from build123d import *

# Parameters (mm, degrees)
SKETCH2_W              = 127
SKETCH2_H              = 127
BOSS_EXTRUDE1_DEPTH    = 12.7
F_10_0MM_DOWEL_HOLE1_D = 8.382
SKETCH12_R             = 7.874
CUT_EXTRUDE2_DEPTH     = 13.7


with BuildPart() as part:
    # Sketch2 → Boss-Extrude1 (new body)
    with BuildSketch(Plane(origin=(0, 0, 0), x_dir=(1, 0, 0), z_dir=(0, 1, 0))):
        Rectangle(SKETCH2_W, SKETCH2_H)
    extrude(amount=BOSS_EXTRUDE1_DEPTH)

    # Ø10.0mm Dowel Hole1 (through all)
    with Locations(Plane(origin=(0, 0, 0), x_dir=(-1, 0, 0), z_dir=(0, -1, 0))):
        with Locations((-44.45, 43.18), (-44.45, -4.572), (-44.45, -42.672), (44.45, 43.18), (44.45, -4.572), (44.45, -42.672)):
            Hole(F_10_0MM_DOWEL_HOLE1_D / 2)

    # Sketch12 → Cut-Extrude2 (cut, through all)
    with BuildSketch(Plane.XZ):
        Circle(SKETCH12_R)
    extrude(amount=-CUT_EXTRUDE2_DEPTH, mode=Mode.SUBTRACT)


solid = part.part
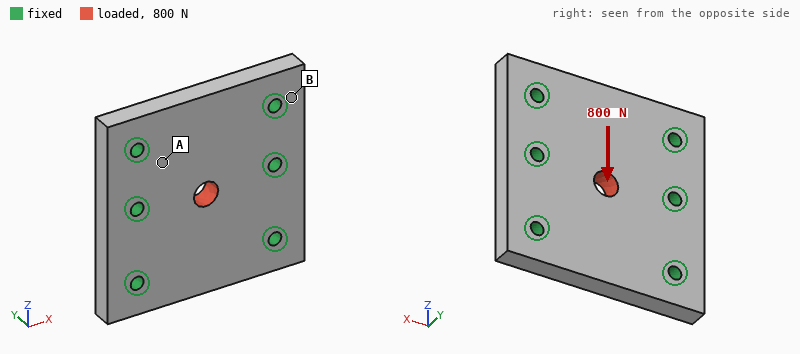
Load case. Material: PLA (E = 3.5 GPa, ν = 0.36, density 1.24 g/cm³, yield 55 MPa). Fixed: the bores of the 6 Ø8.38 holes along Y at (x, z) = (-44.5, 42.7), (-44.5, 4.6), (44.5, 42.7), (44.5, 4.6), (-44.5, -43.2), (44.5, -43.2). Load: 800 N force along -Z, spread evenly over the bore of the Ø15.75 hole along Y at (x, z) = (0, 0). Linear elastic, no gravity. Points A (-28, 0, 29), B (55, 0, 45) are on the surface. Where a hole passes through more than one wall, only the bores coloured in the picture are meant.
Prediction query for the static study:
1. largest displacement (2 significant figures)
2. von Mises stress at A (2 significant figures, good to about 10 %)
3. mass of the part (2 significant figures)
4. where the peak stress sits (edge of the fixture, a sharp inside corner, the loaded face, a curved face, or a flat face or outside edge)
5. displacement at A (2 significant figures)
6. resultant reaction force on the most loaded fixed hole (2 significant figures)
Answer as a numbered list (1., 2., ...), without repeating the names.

1. 13 µm
2. 0.60 MPa
3. 250 g
4. the loaded face
5. 3.7 µm
6. 160 N
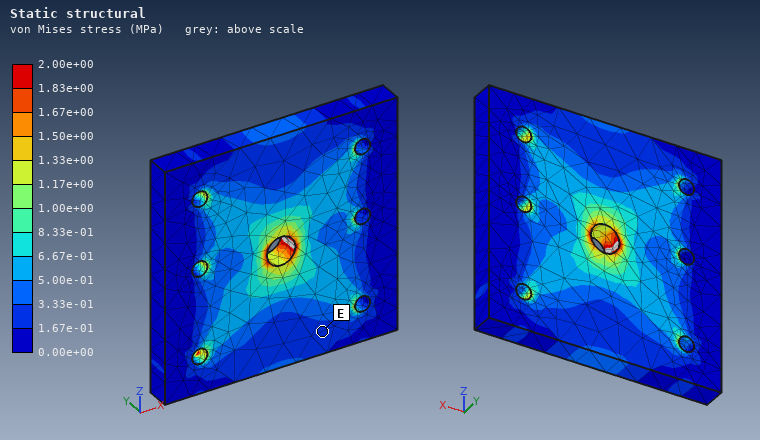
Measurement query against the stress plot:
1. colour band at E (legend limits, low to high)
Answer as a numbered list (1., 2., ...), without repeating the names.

1. 1.67e-01 to 3.33e-01 MPa
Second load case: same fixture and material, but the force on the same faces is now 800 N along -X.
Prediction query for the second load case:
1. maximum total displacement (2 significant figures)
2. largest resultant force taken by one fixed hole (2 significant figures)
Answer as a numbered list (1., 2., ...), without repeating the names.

1. 9.6 µm
2. 230 N
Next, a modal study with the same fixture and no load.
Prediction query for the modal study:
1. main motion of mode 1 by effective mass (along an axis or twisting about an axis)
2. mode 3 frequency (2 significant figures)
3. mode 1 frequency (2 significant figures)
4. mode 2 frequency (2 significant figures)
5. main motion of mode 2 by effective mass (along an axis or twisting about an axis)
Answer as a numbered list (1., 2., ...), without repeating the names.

1. along Y
2. 3200 Hz
3. 2300 Hz
4. 2500 Hz
5. twisting about X
